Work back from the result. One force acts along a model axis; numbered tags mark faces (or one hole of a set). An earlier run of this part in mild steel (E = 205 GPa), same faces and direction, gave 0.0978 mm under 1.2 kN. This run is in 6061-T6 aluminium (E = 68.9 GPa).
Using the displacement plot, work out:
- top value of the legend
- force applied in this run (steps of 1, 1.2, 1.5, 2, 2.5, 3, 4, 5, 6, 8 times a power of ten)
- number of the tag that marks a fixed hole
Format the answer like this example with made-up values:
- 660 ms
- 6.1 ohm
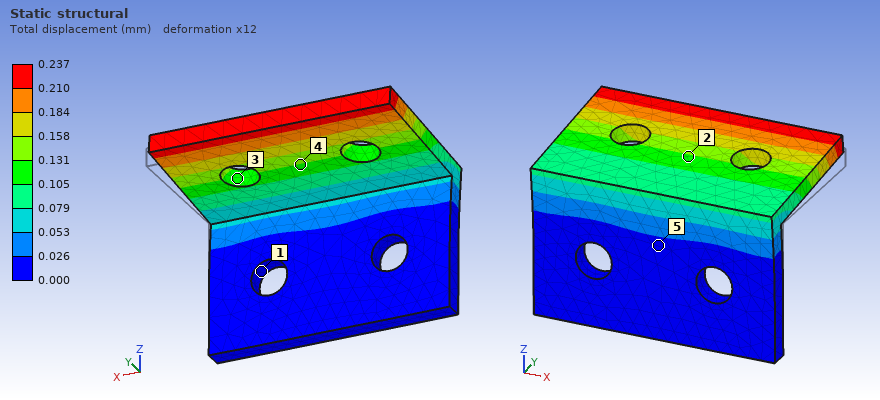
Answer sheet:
- 0.237 mm
- 1 kN
- 1
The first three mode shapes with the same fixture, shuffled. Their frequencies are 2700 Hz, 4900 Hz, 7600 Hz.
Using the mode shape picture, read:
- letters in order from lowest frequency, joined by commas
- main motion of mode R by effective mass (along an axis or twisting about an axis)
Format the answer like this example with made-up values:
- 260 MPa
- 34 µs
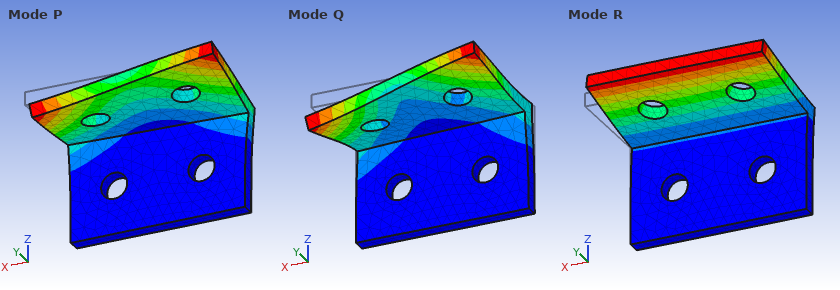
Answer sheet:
- R, P, Q
- along Z
